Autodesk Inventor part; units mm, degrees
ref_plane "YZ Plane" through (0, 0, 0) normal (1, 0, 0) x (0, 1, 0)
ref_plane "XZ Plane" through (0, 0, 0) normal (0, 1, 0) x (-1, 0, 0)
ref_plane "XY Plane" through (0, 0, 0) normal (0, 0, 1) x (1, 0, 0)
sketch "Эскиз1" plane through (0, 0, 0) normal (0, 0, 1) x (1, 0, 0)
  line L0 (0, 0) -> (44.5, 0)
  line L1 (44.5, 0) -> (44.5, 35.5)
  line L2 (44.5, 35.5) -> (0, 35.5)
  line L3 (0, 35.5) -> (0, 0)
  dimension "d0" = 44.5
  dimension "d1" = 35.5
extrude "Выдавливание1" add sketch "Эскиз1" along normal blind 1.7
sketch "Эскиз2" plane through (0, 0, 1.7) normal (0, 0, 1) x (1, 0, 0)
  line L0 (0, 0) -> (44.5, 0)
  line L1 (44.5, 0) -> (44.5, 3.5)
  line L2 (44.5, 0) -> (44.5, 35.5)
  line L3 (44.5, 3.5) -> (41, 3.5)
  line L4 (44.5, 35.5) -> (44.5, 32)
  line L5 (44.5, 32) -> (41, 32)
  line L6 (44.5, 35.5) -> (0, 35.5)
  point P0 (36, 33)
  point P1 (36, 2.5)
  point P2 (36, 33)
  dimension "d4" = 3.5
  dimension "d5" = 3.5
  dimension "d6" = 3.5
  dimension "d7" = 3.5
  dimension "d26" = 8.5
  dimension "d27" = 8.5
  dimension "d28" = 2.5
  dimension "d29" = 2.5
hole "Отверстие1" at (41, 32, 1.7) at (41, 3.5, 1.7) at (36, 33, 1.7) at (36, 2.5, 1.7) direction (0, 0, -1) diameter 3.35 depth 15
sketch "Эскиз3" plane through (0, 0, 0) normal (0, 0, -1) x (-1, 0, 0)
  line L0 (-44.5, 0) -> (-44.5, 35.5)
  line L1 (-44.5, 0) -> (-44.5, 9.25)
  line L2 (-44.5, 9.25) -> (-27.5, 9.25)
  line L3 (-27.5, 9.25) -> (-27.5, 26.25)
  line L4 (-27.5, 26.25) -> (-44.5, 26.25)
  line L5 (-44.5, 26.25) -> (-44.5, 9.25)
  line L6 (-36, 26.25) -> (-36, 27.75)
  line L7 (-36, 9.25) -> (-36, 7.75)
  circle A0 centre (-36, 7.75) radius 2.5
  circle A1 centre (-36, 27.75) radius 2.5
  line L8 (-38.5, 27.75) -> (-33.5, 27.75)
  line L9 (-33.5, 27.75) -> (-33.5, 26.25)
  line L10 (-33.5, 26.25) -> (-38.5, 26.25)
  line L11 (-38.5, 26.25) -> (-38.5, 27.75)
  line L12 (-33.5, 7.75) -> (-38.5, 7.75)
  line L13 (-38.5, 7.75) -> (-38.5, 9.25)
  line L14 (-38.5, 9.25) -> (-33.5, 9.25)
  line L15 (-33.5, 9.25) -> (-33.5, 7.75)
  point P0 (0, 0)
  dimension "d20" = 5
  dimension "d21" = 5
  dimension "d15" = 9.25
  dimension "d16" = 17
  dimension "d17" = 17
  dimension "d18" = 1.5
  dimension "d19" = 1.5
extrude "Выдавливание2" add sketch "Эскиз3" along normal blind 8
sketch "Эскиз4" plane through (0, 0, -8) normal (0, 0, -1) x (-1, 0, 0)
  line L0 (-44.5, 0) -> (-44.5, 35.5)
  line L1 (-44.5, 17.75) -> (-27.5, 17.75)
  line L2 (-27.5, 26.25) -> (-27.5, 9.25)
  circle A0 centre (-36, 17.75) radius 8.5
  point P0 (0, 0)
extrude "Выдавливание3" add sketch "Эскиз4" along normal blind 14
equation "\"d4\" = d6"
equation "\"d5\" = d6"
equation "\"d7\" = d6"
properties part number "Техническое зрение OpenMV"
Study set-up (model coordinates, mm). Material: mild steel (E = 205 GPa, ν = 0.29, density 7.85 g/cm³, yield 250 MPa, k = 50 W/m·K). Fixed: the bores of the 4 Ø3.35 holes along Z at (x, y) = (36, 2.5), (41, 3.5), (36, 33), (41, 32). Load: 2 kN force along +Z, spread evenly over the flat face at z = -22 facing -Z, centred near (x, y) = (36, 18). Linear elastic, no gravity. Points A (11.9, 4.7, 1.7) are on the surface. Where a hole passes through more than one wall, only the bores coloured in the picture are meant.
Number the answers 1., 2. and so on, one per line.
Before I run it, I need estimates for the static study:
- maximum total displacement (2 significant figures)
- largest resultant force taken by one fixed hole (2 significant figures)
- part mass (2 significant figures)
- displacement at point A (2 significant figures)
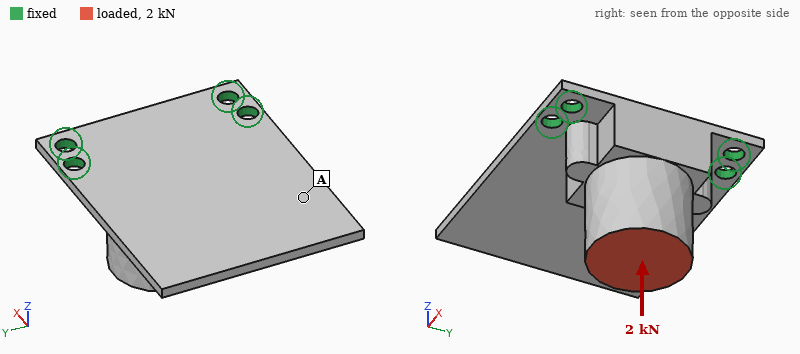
1. 45 µm
2. 930 N
3. 66 g
4. 28 µm
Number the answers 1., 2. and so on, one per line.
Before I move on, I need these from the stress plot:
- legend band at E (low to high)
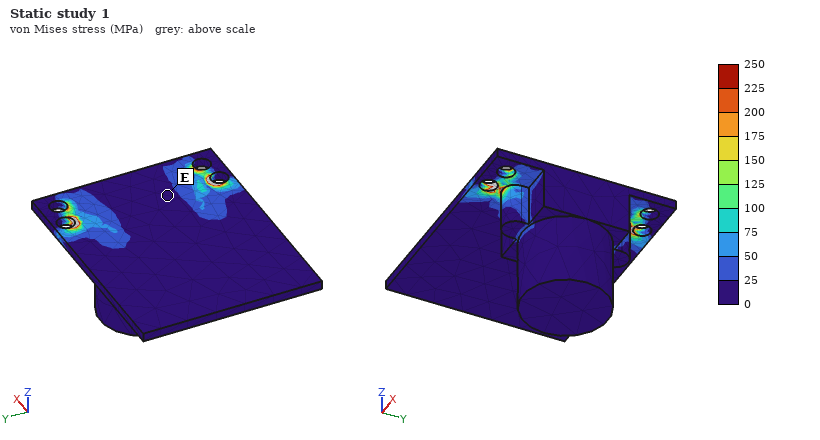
1. 0 to 25 MPa
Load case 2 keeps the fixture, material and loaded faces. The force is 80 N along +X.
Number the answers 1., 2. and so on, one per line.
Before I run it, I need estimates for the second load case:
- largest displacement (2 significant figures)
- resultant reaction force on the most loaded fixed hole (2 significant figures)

1. 24 µm
2. 130 N
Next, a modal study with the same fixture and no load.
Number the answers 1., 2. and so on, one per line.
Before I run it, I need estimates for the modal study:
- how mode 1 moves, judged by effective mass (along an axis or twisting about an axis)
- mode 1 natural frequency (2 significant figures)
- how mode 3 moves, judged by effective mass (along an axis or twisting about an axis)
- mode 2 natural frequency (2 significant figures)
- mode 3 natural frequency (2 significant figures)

1. along Z
2. 1400 Hz
3. along X
4. 3200 Hz
5. 3400 Hz
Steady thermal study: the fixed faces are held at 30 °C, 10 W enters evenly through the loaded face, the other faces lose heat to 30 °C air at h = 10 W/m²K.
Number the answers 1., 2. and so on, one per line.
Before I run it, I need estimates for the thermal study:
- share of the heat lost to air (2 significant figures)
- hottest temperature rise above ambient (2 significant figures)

1. 7.8 %
2. 36 K
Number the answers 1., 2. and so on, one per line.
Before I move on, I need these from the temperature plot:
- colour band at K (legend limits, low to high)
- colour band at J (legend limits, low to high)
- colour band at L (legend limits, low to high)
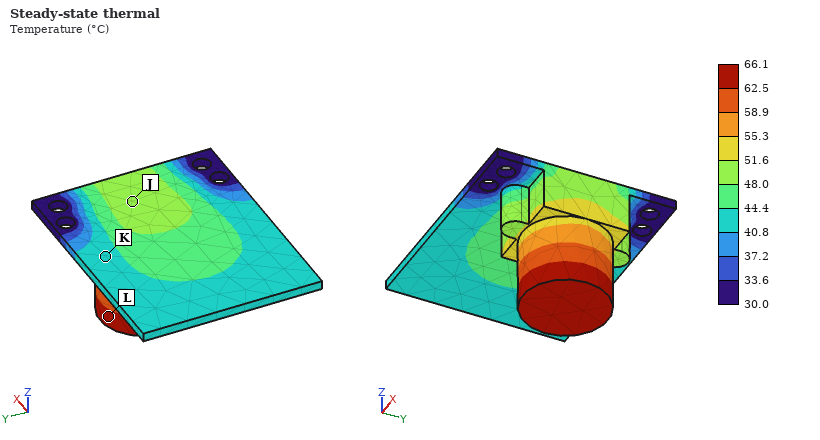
1. 40.8 to 44.4 °C
2. 48.0 to 51.6 °C
3. 62.5 to 66.1 °C
